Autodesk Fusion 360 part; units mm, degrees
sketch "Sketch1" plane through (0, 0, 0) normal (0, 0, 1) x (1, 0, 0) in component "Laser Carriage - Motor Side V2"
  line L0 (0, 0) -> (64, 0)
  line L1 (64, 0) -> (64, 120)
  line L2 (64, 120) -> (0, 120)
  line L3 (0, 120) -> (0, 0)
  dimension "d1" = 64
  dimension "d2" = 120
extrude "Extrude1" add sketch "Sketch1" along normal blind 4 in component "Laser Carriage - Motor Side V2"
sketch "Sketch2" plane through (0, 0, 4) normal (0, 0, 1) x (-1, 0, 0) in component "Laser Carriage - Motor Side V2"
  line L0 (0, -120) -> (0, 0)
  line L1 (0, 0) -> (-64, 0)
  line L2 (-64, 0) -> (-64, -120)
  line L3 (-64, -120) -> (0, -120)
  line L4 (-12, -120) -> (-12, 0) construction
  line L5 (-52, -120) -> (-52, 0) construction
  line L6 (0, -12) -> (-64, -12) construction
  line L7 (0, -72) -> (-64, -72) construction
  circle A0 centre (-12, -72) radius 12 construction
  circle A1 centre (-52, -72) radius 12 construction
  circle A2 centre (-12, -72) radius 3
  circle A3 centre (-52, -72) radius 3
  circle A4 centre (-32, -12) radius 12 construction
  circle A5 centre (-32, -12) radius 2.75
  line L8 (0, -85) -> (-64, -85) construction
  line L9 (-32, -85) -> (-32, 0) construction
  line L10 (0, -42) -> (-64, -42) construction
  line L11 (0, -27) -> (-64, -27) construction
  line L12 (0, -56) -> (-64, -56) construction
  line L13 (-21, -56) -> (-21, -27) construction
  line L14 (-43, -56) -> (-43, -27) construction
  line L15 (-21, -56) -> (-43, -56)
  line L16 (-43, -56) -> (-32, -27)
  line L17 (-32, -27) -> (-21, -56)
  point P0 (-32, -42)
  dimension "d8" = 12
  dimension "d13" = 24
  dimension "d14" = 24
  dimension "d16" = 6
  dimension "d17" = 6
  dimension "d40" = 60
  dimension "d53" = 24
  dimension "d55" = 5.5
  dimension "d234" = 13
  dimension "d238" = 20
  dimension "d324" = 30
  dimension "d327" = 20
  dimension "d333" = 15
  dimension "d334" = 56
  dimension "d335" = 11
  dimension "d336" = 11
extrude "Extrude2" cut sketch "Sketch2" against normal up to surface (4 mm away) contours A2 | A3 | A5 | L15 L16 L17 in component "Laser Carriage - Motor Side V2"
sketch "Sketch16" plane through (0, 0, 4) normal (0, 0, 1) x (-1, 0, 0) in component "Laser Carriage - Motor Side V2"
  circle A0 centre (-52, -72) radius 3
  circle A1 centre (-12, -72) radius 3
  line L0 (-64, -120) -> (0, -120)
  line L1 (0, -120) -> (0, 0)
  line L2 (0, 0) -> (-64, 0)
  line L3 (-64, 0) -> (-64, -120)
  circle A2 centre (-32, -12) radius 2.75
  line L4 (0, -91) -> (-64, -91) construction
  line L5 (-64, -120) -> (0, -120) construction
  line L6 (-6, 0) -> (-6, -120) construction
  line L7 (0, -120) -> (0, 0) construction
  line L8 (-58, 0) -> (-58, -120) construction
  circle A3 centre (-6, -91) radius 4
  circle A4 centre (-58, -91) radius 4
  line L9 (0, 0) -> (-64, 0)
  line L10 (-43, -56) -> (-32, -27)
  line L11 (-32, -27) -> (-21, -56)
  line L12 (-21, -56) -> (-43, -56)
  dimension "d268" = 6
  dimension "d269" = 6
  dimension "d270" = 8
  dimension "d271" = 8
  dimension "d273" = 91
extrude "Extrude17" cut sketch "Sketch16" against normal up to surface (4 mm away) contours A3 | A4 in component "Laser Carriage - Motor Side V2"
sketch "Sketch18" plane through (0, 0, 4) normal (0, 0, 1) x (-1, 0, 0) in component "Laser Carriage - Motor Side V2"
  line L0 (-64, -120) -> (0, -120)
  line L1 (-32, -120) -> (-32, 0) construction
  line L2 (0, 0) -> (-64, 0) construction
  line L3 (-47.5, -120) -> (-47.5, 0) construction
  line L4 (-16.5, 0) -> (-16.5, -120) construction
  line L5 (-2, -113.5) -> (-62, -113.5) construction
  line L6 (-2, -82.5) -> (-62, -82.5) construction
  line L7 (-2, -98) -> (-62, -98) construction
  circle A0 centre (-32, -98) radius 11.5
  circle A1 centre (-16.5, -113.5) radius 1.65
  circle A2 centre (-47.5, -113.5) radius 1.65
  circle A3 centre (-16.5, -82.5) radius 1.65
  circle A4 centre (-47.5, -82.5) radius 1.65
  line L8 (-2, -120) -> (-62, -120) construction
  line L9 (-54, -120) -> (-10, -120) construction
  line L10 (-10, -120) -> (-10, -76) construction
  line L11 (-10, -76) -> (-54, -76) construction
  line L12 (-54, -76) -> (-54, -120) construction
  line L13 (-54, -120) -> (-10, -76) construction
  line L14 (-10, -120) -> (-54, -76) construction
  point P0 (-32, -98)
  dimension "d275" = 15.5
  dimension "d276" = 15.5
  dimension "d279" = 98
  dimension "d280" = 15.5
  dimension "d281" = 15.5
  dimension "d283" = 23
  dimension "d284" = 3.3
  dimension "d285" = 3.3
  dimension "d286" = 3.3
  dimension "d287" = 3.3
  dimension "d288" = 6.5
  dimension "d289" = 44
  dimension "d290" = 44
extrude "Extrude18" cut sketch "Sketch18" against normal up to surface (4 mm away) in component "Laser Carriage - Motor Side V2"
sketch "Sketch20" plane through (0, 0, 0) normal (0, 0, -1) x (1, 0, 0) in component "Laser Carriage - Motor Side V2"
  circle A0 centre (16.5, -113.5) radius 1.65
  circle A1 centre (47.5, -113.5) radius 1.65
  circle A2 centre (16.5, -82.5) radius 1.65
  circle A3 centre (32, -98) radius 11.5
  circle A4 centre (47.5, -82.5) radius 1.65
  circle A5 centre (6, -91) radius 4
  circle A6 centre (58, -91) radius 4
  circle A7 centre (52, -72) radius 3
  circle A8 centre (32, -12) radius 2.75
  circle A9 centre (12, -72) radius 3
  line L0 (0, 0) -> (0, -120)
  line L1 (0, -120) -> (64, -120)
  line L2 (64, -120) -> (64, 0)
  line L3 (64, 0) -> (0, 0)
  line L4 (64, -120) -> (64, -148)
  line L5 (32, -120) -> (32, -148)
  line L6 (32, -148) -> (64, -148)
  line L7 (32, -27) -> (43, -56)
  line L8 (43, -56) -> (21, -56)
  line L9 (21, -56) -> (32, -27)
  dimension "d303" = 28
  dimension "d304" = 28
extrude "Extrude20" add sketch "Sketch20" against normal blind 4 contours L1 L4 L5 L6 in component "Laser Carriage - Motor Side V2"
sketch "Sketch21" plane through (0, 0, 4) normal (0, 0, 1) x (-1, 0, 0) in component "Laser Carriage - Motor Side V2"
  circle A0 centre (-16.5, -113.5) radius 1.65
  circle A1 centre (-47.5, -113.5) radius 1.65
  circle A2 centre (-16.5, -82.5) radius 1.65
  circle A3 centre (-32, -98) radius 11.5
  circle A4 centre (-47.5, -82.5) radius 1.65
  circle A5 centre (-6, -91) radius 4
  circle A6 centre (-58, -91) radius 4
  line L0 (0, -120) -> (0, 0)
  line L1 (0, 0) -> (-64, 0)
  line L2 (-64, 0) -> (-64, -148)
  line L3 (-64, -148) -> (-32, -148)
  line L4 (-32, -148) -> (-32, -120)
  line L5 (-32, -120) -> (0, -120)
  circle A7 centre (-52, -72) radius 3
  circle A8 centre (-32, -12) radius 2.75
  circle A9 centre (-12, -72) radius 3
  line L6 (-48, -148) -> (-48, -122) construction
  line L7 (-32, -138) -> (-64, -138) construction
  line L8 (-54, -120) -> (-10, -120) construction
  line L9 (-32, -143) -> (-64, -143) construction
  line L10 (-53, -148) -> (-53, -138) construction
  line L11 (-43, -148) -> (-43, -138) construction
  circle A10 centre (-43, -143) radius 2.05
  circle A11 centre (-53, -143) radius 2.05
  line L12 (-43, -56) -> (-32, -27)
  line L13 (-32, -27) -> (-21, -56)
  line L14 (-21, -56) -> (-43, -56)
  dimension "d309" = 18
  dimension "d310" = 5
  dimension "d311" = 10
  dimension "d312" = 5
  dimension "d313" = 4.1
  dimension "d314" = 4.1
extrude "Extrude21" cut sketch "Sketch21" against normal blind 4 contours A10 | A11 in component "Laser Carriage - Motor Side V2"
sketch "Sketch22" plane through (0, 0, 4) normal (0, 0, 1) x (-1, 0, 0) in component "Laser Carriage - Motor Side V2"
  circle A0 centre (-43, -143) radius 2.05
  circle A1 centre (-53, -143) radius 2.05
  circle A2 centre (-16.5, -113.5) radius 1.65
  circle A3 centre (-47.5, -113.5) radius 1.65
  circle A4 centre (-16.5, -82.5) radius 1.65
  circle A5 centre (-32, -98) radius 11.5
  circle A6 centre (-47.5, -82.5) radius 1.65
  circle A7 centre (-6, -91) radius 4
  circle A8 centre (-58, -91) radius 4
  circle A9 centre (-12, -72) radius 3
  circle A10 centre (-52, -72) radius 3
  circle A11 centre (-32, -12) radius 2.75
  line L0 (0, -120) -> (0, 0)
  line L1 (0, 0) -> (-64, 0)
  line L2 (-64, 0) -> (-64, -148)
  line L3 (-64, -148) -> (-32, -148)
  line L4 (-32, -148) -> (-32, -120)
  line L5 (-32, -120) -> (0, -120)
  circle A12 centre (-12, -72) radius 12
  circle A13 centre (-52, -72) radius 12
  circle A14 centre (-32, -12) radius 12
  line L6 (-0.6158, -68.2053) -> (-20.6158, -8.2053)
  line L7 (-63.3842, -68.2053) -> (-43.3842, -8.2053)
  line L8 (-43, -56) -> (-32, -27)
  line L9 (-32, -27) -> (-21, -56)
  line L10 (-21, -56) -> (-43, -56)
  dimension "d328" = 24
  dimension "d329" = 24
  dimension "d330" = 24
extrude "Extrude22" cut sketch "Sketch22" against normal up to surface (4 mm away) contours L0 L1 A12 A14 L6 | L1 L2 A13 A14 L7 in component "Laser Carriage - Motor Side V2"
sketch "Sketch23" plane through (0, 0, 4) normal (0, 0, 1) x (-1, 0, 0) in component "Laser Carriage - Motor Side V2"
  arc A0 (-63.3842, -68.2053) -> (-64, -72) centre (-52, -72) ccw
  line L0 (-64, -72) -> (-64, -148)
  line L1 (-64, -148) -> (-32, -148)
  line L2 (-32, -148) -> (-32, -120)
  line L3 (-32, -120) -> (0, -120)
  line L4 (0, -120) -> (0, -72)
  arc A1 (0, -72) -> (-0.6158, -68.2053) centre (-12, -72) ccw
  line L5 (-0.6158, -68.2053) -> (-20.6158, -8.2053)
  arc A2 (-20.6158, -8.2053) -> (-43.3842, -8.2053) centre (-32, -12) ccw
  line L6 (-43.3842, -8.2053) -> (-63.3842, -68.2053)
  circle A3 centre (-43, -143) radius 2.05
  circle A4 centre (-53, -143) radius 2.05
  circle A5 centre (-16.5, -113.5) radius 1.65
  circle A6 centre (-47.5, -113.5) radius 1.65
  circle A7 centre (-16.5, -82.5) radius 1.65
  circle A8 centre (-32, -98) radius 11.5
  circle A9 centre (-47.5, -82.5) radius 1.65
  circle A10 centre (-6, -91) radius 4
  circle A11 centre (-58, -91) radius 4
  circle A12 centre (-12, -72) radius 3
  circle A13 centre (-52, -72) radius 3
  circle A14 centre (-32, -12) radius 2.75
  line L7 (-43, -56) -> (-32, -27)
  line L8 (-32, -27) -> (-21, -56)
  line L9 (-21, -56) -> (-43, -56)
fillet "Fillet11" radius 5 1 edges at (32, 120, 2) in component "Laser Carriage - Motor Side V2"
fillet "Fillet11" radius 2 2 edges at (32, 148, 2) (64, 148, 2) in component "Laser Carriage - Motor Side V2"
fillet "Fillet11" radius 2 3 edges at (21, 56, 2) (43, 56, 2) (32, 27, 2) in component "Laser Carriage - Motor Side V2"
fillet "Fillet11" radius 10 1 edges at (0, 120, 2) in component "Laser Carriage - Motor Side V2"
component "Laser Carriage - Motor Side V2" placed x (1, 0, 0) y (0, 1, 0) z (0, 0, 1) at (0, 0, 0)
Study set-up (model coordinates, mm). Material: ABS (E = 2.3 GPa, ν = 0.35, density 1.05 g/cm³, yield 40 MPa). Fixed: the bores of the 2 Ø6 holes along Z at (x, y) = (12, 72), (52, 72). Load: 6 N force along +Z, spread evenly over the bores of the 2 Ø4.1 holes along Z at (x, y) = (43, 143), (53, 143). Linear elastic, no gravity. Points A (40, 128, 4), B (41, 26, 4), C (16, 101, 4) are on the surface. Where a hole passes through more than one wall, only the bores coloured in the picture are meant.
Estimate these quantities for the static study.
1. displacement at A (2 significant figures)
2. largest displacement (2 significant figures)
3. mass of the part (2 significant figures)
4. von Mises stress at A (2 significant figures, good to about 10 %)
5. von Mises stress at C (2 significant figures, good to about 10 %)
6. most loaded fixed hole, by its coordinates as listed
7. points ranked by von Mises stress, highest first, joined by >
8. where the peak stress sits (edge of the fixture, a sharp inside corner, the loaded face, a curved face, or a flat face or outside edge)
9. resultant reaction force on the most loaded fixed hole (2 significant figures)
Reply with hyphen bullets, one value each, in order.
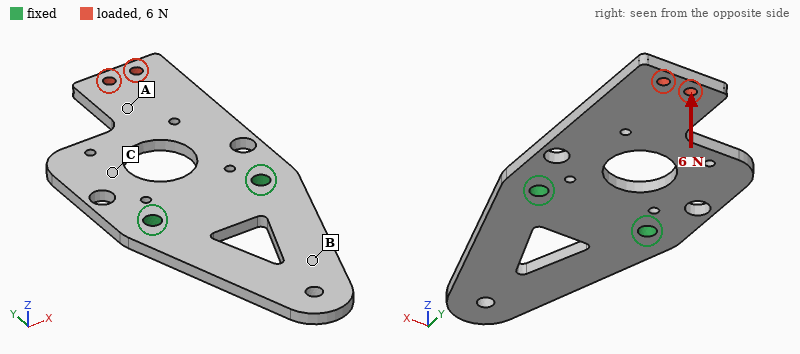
- 0.98 mm
- 1.8 mm
- 25 g
- 1.4 MPa
- 2.4 MPa
- (52, 72)
- C > A > B
- a curved face
- 4.9 N
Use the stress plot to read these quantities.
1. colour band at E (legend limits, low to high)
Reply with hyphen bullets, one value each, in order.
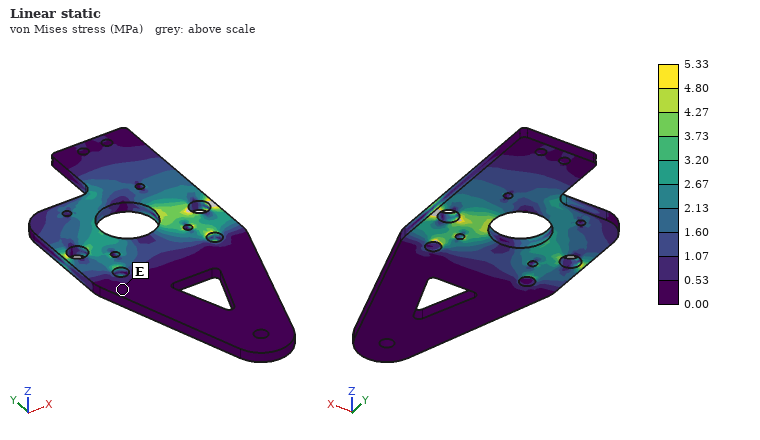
- 0.00 to 0.53 MPa
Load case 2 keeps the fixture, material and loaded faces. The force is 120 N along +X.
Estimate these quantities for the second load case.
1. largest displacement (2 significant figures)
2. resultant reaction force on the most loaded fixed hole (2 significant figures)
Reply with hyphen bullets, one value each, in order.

- 0.37 mm
- 210 N
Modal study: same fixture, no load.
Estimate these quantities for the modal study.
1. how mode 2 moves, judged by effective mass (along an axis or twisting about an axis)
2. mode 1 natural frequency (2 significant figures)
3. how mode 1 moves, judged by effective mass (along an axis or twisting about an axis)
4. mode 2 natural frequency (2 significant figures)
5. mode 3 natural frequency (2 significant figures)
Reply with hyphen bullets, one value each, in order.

- along Z
- 180 Hz
- along Z
- 250 Hz
- 610 Hz
